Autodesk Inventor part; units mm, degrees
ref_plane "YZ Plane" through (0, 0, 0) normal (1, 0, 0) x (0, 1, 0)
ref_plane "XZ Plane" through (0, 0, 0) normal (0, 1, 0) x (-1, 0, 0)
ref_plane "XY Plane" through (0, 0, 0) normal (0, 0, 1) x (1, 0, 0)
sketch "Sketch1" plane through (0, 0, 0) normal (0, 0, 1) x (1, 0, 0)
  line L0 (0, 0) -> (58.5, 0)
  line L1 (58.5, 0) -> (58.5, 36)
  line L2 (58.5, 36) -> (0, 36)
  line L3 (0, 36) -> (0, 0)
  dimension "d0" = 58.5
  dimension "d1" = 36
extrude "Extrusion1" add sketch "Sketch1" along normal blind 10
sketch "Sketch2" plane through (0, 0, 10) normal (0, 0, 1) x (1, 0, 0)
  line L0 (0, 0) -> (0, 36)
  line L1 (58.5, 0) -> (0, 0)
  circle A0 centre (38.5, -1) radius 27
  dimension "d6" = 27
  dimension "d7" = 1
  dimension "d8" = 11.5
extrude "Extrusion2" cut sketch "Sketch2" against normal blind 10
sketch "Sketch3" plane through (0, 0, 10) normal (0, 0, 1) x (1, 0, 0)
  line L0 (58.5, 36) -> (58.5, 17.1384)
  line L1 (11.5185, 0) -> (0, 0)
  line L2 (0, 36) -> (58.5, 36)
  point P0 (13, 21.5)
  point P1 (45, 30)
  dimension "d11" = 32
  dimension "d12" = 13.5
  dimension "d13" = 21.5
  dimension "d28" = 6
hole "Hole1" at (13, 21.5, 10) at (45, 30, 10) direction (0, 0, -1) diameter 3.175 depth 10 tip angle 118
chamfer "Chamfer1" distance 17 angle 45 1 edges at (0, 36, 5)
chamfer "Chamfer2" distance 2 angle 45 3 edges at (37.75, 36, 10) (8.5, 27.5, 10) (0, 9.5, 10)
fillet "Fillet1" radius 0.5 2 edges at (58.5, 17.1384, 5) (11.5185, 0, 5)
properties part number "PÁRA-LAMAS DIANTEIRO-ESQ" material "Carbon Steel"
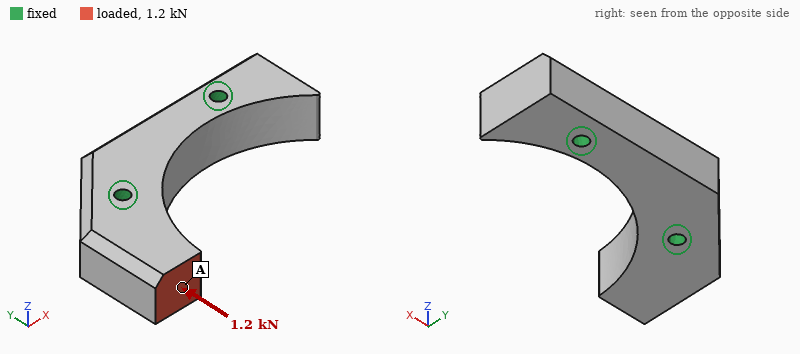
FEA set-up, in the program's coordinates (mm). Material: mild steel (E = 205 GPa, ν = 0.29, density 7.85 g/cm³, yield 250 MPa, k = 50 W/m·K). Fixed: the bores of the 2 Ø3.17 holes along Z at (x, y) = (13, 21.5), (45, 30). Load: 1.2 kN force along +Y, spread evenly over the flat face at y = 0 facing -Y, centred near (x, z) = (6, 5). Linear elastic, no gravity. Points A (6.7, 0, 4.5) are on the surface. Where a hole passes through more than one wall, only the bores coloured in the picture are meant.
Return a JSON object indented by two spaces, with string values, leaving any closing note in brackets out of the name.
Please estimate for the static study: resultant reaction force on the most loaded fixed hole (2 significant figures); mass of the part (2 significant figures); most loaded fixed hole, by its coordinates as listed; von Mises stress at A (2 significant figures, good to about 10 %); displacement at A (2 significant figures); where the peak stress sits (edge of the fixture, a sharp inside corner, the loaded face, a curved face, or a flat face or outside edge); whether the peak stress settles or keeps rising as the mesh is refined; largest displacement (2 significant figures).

{
  "resultant reaction force on the most loaded fixed hole": "1.3 kN",
  "mass of the part": "72 g",
  "most loaded fixed hole, by its coordinates as listed": "(13, 21.5)",
  "von Mises stress at A": "9.9 MPa",
  "displacement at A": "6.0 µm",
  "where the peak stress sits": "edge of the fixture",
  "whether the peak stress settles or keeps rising as the mesh is refined": "keeps rising",
  "largest displacement": "7.1 µm"
}
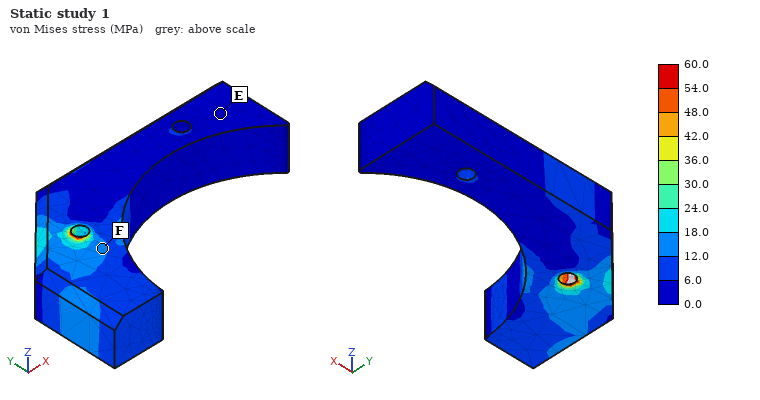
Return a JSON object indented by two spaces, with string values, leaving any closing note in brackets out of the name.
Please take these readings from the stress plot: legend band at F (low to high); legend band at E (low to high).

{
  "legend band at F": "12.0 to 18.0 MPa",
  "legend band at E": "0.0 to 6.0 MPa"
}
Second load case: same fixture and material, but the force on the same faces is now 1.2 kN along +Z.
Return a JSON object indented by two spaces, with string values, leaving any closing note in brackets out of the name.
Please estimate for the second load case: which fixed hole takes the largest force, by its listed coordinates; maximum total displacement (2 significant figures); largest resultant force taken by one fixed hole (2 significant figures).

{
  "which fixed hole takes the largest force, by its listed coordinates": "(13, 21.5)",
  "maximum total displacement": "29 µm",
  "largest resultant force taken by one fixed hole": "1.3 kN"
}
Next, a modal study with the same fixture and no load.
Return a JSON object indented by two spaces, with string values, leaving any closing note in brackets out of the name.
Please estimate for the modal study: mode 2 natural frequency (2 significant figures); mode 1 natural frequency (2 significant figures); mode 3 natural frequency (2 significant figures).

{
  "mode 2 natural frequency": "14 kHz",
  "mode 1 natural frequency": "14 kHz",
  "mode 3 natural frequency": "21 kHz"
}
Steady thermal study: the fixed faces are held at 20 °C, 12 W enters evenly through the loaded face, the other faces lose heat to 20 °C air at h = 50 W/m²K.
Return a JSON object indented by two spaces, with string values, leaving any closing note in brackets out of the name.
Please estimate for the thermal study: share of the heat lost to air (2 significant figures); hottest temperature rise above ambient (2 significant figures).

{
  "share of the heat lost to air": "9.1 %",
  "hottest temperature rise above ambient": "41 K"
}
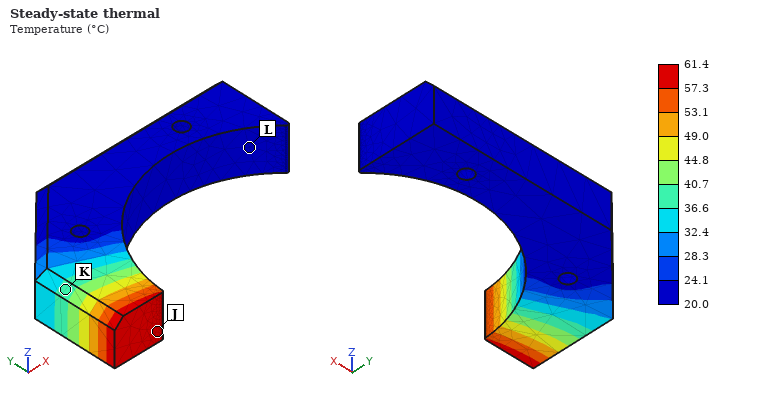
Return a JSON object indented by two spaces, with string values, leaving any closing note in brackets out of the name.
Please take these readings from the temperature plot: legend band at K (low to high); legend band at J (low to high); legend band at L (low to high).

{
  "legend band at K": "36.6 to 40.7 °C",
  "legend band at J": "57.3 to 61.4 °C",
  "legend band at L": "20.0 to 24.1 °C"
}
